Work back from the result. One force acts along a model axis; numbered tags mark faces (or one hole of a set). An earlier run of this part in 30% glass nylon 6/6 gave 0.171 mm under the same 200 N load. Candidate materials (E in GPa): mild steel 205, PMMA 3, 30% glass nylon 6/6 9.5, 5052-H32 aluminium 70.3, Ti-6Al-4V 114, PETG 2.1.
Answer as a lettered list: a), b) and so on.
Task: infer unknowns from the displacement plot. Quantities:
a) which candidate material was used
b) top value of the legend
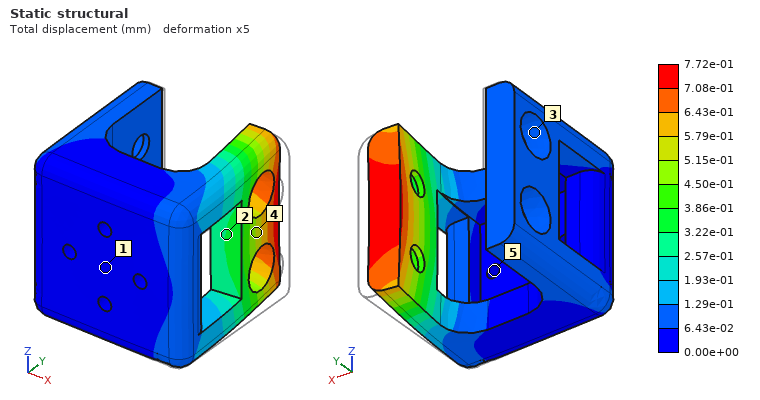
a) PETG
b) 7.72e-01 mm
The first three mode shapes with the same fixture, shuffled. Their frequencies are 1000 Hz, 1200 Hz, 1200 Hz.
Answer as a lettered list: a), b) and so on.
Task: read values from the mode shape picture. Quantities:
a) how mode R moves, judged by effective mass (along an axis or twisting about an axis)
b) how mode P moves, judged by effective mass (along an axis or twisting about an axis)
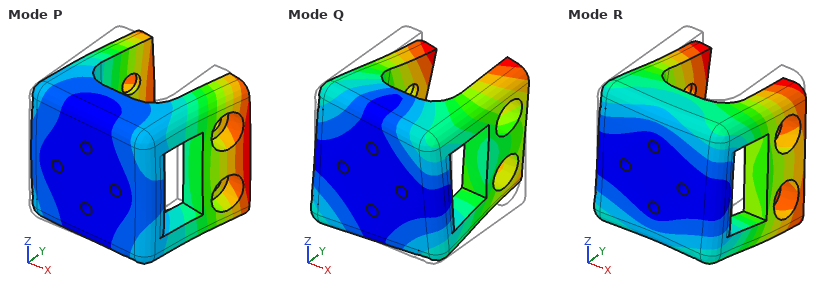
a) along Z
b) along X
